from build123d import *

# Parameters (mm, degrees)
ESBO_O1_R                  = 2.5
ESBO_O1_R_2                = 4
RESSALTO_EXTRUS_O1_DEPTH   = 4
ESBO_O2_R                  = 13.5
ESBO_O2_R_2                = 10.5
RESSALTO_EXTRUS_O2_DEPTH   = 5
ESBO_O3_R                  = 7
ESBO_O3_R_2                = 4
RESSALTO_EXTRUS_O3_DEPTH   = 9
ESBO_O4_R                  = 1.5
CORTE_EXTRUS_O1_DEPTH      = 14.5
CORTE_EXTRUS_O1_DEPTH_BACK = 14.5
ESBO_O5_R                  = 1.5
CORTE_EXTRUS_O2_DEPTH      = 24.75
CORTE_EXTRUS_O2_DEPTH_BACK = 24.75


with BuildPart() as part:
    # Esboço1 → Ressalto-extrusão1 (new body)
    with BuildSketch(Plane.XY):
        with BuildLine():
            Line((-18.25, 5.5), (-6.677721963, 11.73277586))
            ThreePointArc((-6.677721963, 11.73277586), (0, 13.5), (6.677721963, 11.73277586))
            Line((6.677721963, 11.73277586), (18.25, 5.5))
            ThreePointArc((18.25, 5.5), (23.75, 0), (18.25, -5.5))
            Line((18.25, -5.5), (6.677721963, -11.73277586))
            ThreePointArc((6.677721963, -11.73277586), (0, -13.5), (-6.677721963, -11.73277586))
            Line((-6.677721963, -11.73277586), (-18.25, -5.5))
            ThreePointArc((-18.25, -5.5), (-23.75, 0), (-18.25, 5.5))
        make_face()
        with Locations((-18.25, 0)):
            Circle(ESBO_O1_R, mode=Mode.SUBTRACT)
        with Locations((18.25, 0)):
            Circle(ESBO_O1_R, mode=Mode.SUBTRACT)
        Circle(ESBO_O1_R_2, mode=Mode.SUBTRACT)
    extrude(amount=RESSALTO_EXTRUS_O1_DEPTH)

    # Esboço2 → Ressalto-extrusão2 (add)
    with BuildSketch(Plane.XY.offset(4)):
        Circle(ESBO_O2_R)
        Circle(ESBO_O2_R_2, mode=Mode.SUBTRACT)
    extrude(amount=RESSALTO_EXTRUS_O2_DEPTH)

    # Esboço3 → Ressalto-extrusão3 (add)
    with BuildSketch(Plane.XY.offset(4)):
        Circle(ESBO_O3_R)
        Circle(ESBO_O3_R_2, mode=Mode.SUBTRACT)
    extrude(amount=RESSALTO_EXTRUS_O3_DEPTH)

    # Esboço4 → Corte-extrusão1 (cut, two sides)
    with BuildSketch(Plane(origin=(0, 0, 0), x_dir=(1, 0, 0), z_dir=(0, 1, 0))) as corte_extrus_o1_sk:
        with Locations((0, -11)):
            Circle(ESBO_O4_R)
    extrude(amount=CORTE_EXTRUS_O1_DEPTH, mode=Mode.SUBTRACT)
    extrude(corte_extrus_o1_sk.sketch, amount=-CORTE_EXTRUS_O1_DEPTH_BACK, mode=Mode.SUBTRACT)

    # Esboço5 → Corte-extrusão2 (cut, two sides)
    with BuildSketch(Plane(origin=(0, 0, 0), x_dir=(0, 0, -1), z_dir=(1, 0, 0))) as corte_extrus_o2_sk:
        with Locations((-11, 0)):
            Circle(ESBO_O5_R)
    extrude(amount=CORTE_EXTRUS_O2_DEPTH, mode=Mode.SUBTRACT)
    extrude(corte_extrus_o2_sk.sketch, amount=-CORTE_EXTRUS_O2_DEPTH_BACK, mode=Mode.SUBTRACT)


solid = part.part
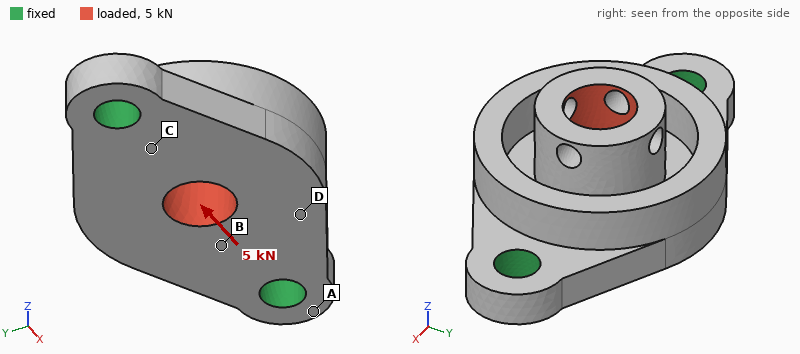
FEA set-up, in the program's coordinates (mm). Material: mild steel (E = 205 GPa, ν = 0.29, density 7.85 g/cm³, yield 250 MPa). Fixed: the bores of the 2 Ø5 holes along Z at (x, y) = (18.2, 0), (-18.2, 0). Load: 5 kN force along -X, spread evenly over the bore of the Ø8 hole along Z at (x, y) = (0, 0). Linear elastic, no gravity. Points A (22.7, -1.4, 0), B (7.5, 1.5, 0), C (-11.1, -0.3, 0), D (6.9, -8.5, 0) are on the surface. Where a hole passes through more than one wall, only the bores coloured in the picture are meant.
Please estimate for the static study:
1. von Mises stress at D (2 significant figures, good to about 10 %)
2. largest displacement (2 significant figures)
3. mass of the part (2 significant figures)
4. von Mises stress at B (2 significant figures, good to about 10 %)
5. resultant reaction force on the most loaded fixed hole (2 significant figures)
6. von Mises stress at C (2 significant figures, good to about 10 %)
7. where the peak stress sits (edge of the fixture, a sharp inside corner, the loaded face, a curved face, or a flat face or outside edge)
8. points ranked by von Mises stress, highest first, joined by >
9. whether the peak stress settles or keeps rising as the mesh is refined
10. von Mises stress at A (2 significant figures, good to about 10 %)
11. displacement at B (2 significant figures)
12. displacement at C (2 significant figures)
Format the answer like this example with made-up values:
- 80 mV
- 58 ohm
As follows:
- 20 MPa
- 16 µm
- 39 g
- 41 MPa
- 2.6 kN
- 55 MPa
- edge of the fixture
- C > B > D > A
- keeps rising
- 13 MPa
- 4.3 µm
- 3.2 µm
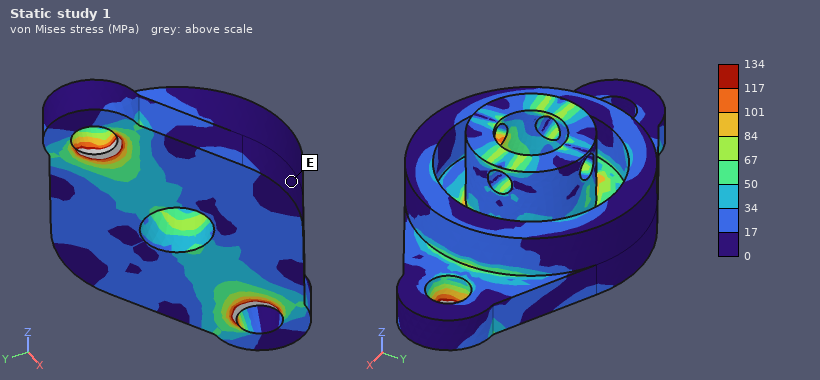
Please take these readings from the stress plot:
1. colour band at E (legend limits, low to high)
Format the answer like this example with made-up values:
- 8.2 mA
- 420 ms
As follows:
- 0 to 17 MPa
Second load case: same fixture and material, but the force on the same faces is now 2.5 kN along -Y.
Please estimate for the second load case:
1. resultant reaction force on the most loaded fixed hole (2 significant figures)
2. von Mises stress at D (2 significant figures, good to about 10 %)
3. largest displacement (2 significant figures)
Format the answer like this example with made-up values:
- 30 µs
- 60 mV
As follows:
- 1.3 kN
- 38 MPa
- 25 µm
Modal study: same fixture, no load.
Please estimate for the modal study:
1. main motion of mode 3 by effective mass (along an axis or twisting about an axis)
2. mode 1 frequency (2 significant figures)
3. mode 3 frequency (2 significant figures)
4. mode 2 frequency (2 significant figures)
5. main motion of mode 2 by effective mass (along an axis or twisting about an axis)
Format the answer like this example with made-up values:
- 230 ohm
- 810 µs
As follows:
- along Y
- 9700 Hz
- 27 kHz
- 13 kHz
- along Z
